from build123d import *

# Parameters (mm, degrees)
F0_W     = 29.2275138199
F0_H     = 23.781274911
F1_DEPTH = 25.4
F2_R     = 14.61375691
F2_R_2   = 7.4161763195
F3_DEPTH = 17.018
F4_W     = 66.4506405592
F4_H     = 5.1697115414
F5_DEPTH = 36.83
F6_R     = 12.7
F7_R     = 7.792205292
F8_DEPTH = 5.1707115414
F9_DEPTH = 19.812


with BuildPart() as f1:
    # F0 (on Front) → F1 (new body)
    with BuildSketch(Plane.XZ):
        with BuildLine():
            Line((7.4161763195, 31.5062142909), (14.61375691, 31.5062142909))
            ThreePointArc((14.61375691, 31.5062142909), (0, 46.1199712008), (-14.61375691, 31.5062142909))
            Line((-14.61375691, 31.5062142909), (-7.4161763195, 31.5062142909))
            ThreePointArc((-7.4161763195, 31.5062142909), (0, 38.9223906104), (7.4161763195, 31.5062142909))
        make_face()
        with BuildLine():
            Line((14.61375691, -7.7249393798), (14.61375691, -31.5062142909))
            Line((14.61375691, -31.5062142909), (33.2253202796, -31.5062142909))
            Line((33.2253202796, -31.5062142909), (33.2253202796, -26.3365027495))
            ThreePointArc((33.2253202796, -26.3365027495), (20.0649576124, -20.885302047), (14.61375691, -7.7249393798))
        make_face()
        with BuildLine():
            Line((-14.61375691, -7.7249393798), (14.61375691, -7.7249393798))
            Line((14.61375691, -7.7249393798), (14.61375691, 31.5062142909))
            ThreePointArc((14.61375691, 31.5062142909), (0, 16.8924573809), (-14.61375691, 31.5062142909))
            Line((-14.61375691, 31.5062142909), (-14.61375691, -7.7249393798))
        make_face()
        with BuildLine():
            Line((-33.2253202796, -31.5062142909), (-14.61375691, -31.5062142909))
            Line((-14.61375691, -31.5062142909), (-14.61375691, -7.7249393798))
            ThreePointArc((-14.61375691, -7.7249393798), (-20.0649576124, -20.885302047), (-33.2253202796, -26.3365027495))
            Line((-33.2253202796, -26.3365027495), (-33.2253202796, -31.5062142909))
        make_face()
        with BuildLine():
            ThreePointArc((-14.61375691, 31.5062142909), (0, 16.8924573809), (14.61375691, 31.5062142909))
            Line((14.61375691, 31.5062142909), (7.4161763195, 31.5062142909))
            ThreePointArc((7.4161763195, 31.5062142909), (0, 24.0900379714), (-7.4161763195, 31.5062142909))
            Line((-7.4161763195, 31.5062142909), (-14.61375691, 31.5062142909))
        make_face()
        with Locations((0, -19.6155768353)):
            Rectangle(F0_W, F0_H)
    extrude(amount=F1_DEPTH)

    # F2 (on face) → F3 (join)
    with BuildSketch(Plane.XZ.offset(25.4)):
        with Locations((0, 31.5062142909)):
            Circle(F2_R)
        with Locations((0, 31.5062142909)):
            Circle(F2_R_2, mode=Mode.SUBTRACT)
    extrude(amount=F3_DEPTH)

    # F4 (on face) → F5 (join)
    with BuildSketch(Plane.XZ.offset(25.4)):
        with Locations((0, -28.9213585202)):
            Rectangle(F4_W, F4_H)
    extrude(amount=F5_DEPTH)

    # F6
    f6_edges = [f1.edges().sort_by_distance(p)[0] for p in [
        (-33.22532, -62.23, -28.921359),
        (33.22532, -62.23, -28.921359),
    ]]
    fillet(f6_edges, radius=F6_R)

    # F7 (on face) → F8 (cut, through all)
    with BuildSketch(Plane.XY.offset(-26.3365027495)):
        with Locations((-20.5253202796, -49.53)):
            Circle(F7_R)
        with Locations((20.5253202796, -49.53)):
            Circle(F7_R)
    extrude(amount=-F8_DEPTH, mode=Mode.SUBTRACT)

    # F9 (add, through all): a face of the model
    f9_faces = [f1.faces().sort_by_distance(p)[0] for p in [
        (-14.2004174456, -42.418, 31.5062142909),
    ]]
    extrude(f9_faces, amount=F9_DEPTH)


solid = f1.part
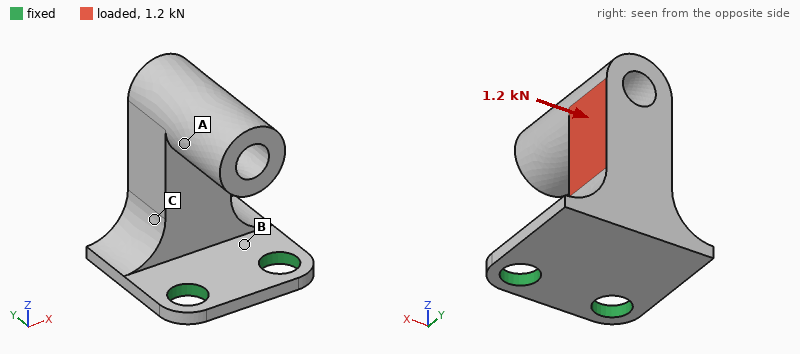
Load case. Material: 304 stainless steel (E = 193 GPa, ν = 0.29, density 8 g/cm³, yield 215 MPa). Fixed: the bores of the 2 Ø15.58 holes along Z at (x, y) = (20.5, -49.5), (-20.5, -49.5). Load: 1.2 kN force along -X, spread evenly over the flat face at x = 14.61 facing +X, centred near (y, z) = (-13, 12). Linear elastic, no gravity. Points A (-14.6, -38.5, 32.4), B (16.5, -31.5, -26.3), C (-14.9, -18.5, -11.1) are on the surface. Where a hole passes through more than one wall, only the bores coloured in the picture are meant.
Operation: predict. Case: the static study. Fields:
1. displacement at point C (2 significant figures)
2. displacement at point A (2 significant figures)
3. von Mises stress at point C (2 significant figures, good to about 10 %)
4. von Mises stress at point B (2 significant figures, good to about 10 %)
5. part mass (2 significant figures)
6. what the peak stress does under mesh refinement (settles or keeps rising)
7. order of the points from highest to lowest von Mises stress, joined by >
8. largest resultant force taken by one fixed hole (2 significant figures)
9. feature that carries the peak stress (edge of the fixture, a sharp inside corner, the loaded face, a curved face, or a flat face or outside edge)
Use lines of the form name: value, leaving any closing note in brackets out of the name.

displacement at point C: 22 µm
displacement at point A: 62 µm
von Mises stress at point C: 15 MPa
von Mises stress at point B: 40 MPa
part mass: 710 g
what the peak stress does under mesh refinement: keeps rising
order of the points from highest to lowest von Mises stress, joined by >: B > C > A
largest resultant force taken by one fixed hole: 1.5 kN
feature that carries the peak stress: edge of the fixture
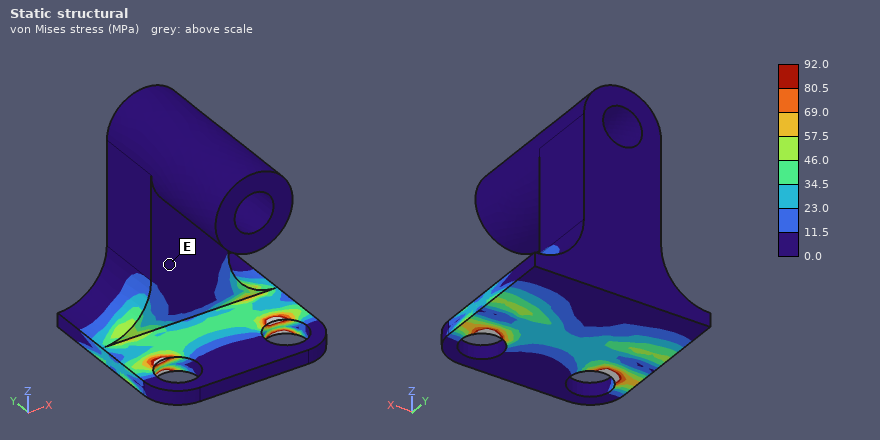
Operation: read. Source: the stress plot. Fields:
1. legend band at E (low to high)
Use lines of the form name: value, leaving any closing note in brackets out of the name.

legend band at E: 0.0 to 11.5 MPa
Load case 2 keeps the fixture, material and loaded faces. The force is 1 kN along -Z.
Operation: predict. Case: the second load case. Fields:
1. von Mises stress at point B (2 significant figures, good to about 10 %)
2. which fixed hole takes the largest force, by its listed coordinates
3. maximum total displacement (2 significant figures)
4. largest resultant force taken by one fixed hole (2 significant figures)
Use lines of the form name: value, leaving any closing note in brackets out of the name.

von Mises stress at point B: 57 MPa
which fixed hole takes the largest force, by its listed coordinates: (20.5, -49.5)
maximum total displacement: 0.24 mm
largest resultant force taken by one fixed hole: 830 N
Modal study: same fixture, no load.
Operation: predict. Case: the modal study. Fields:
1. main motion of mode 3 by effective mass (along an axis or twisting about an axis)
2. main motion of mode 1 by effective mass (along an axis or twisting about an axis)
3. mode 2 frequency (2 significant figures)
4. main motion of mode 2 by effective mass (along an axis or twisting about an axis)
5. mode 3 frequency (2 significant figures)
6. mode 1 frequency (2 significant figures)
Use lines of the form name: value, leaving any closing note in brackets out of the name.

main motion of mode 3 by effective mass: along Z
main motion of mode 1 by effective mass: along Y
mode 2 frequency: 990 Hz
main motion of mode 2 by effective mass: along X
mode 3 frequency: 2200 Hz
mode 1 frequency: 360 Hz
